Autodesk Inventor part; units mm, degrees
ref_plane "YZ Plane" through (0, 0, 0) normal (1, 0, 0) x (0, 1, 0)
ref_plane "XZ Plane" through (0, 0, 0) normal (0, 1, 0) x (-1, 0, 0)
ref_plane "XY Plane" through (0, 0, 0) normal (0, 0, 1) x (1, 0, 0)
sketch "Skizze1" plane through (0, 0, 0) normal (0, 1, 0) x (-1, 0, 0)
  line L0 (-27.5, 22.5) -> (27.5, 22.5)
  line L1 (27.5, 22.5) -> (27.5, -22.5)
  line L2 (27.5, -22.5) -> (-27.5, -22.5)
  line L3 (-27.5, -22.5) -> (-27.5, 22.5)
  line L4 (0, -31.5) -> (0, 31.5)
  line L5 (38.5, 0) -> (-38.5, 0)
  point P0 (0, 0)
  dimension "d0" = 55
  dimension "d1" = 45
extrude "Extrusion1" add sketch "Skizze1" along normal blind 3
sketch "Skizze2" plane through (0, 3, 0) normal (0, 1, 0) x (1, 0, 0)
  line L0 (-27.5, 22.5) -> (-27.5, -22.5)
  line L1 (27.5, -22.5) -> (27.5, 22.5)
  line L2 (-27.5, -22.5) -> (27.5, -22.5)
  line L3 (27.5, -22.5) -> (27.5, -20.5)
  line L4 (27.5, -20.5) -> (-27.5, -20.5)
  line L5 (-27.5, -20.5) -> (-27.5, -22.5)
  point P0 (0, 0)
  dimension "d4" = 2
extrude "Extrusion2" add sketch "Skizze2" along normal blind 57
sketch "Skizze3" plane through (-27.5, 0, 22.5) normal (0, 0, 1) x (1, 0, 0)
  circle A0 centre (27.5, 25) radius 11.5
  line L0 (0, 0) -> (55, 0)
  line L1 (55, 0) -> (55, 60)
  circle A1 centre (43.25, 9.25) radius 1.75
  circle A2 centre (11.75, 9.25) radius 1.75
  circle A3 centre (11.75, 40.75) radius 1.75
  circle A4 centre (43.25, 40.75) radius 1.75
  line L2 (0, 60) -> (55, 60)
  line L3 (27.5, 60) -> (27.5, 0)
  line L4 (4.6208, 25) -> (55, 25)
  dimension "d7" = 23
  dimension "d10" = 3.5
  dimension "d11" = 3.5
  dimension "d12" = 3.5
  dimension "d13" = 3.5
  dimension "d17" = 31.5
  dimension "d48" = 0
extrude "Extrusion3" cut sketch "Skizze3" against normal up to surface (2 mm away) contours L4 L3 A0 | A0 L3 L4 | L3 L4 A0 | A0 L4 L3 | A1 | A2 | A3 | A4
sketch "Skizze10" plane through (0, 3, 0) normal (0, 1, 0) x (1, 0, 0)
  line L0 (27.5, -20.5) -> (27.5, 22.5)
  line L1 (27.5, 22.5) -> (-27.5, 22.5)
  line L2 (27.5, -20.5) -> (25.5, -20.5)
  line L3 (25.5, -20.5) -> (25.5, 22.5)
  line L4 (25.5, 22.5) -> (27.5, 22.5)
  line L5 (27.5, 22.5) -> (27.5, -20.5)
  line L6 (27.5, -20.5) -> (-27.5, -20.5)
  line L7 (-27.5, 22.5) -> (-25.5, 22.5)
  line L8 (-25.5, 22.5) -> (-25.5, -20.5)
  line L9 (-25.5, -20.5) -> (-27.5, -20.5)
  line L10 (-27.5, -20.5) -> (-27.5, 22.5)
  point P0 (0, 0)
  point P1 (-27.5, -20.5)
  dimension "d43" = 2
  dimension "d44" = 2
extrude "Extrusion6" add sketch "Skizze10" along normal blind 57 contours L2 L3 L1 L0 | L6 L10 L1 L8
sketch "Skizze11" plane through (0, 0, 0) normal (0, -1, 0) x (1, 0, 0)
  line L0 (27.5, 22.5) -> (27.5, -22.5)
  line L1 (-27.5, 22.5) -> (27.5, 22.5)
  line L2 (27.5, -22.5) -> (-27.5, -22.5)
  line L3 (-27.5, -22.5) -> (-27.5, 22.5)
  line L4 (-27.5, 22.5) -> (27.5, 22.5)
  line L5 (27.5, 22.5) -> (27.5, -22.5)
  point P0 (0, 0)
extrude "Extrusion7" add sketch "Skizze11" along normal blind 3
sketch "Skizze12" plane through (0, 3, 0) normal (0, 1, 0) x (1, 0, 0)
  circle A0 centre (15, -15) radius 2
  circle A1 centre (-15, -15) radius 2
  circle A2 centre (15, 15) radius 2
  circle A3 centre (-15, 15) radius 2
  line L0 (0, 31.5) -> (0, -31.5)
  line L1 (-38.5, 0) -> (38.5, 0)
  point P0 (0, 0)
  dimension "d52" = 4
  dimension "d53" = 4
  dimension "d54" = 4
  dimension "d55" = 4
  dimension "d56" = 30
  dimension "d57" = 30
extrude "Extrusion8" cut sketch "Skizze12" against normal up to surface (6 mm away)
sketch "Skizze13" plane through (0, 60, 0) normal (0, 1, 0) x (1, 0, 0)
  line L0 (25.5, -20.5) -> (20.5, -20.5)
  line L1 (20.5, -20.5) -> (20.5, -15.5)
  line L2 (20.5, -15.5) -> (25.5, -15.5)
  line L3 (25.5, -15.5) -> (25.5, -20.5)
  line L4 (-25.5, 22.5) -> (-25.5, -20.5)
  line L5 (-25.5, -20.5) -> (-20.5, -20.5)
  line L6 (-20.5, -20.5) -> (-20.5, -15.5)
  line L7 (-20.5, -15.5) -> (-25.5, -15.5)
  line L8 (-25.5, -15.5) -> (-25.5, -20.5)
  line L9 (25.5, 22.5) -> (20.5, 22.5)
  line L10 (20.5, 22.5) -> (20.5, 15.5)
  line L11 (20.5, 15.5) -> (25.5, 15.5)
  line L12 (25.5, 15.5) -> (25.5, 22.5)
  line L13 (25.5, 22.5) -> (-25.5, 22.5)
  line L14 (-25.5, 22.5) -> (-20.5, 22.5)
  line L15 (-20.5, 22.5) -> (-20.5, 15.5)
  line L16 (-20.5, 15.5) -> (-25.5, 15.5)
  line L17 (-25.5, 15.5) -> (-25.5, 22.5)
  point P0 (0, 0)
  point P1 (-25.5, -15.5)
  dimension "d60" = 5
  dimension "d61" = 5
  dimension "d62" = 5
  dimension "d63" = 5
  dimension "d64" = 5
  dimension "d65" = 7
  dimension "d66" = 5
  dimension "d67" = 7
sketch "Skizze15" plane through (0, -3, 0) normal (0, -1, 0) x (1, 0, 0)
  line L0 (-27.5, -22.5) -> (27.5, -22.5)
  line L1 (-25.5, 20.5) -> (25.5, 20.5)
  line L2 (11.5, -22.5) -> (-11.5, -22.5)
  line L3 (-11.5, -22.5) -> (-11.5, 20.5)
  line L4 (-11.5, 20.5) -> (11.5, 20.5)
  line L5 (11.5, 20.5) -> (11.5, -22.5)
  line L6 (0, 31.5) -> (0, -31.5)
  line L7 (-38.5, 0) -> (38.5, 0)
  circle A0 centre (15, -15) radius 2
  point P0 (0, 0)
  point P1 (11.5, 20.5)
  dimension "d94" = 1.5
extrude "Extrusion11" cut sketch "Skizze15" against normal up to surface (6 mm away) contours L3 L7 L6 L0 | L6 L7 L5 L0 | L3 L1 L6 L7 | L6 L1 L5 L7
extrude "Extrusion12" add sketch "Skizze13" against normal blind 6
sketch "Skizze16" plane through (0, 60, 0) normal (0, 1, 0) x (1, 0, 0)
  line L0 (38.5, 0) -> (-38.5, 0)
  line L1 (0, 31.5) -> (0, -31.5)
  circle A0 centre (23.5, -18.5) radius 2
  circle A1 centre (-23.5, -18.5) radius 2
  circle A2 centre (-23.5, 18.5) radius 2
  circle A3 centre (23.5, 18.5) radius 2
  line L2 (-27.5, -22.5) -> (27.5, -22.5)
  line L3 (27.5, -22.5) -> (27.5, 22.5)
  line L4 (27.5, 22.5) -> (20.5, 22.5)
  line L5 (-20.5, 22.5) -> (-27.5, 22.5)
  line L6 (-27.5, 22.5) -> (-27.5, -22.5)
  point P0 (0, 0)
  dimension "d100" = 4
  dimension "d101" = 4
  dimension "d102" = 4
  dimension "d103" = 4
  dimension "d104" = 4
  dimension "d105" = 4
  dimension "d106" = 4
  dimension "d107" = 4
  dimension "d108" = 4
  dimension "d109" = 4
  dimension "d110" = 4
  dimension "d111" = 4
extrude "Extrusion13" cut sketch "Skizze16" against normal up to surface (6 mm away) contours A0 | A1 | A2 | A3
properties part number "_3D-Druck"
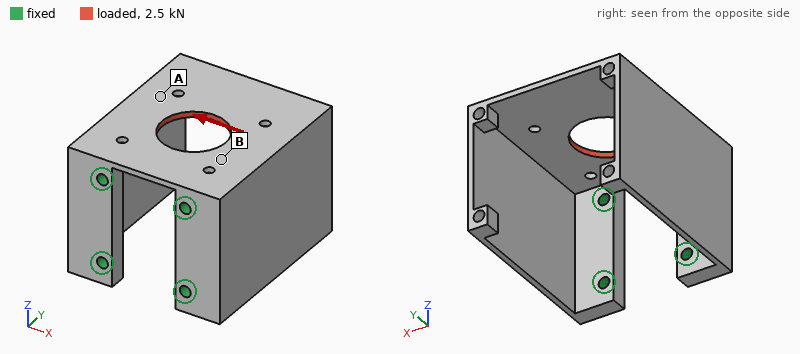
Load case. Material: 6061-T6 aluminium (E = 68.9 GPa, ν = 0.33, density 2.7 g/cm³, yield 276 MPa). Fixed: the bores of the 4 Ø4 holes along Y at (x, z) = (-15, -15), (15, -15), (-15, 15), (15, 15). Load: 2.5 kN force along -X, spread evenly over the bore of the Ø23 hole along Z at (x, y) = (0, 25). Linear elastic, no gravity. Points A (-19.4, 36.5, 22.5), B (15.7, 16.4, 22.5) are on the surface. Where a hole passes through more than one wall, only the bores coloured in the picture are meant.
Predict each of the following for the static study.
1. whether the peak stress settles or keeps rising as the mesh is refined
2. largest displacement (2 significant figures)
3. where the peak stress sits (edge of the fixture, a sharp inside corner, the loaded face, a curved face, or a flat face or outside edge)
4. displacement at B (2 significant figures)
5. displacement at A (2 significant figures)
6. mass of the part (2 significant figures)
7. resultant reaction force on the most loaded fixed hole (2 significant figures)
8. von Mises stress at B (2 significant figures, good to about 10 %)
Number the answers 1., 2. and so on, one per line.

1. keeps rising
2. 0.15 mm
3. edge of the fixture
4. 0.049 mm
5. 0.10 mm
6. 65 g
7. 2.1 kN
8. 49 MPa
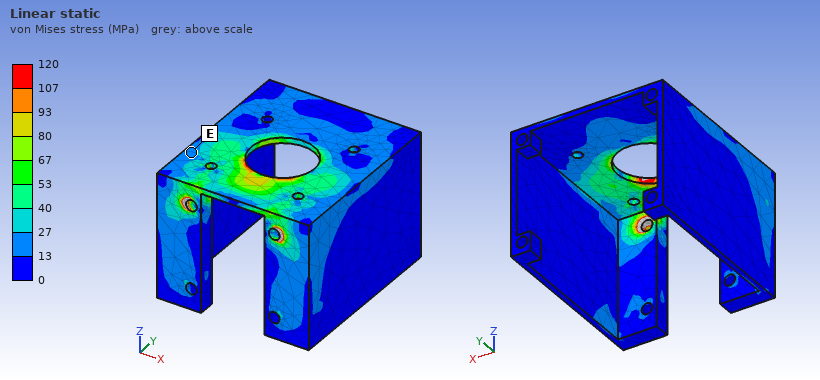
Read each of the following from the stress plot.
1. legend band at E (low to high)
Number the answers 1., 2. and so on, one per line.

1. 13 to 27 MPa
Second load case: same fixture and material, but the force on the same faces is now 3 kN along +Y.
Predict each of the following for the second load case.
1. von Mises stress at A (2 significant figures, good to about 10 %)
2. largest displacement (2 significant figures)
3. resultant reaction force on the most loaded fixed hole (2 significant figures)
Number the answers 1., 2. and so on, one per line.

1. 11 MPa
2. 48 µm
3. 1.6 kN
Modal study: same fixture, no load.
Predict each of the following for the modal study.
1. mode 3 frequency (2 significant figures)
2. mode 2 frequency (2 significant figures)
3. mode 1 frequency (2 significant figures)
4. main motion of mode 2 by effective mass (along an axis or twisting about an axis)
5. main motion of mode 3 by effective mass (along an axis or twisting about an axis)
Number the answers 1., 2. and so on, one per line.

1. 2800 Hz
2. 1100 Hz
3. 970 Hz
4. along X
5. along Z
